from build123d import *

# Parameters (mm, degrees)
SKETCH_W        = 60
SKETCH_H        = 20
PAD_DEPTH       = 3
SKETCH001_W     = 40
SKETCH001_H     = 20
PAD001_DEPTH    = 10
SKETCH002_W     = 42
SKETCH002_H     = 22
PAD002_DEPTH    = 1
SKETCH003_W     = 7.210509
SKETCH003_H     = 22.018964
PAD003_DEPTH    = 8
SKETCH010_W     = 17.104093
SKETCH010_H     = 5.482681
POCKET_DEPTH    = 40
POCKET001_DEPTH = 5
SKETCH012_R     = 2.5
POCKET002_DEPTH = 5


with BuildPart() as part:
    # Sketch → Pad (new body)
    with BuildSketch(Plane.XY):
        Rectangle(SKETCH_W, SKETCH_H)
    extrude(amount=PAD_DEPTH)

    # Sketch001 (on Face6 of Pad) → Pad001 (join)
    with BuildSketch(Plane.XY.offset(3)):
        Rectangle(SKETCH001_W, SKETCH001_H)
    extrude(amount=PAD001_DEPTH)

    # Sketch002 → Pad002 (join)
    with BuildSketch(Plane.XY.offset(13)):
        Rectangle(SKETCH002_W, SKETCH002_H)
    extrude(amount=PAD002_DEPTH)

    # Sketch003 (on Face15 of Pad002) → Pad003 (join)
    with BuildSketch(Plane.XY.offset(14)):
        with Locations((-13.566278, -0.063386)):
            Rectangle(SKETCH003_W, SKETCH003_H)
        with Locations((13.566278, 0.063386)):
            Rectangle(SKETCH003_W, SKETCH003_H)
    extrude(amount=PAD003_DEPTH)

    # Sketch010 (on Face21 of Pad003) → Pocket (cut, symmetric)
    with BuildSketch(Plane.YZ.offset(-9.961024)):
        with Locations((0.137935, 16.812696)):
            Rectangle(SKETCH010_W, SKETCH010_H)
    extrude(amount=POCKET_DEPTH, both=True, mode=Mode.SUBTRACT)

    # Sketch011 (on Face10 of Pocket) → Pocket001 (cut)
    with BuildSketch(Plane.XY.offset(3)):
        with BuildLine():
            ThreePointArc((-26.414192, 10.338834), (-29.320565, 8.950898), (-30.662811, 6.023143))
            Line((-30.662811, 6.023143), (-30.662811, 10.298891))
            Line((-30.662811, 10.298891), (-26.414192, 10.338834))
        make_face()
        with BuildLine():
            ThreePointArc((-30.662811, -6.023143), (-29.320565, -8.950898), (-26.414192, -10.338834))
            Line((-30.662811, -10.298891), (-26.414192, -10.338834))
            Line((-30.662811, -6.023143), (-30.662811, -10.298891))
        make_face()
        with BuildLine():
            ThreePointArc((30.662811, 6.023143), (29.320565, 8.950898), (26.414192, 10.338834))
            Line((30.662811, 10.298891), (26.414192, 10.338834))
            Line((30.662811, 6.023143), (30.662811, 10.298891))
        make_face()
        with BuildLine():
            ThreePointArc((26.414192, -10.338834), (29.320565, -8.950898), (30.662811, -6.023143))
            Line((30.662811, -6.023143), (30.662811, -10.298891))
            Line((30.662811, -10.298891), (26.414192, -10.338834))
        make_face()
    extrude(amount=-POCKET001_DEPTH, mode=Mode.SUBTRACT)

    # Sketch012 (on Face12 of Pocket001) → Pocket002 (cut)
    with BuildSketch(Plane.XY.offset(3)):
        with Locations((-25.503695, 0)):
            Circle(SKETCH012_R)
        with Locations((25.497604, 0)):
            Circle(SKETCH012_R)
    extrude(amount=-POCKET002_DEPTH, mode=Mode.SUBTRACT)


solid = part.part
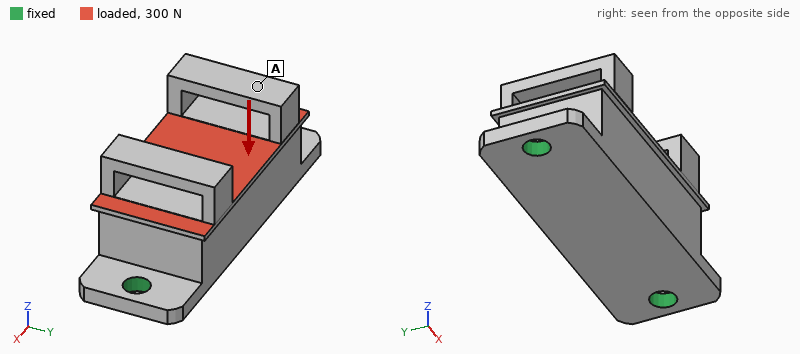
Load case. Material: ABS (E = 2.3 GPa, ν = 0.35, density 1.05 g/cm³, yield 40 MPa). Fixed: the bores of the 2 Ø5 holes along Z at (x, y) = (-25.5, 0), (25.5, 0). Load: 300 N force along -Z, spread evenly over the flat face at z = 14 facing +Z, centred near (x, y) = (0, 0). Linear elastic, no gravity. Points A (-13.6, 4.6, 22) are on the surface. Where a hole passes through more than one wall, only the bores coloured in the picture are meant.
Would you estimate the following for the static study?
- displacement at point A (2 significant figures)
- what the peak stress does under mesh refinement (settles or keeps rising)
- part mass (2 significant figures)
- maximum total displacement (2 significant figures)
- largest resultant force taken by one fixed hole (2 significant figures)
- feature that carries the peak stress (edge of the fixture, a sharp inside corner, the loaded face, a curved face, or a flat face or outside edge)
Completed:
73 µm
keeps rising
14 g
87 µm
180 N
edge of the fixture
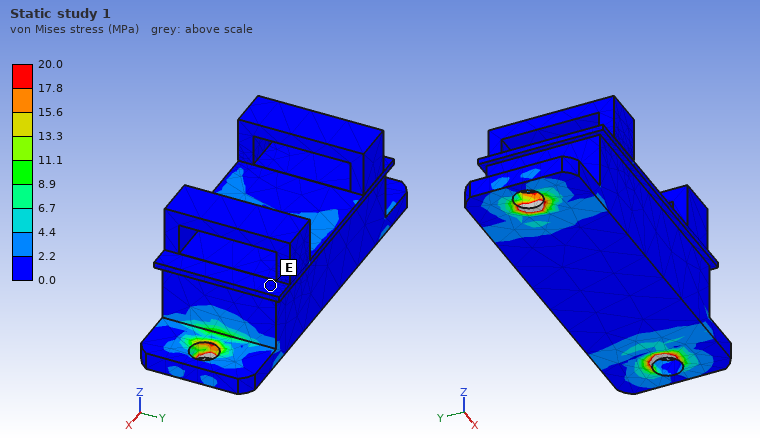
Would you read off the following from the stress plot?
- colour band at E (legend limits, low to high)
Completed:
0.0 to 2.2 MPa
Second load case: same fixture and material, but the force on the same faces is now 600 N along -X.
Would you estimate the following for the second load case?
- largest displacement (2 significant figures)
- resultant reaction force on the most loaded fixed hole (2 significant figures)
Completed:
98 µm
350 N
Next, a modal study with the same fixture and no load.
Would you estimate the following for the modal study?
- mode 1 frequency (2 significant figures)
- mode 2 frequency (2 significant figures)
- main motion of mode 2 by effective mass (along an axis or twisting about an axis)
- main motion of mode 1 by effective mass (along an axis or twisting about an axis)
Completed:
1200 Hz
2800 Hz
along Z
along Y
